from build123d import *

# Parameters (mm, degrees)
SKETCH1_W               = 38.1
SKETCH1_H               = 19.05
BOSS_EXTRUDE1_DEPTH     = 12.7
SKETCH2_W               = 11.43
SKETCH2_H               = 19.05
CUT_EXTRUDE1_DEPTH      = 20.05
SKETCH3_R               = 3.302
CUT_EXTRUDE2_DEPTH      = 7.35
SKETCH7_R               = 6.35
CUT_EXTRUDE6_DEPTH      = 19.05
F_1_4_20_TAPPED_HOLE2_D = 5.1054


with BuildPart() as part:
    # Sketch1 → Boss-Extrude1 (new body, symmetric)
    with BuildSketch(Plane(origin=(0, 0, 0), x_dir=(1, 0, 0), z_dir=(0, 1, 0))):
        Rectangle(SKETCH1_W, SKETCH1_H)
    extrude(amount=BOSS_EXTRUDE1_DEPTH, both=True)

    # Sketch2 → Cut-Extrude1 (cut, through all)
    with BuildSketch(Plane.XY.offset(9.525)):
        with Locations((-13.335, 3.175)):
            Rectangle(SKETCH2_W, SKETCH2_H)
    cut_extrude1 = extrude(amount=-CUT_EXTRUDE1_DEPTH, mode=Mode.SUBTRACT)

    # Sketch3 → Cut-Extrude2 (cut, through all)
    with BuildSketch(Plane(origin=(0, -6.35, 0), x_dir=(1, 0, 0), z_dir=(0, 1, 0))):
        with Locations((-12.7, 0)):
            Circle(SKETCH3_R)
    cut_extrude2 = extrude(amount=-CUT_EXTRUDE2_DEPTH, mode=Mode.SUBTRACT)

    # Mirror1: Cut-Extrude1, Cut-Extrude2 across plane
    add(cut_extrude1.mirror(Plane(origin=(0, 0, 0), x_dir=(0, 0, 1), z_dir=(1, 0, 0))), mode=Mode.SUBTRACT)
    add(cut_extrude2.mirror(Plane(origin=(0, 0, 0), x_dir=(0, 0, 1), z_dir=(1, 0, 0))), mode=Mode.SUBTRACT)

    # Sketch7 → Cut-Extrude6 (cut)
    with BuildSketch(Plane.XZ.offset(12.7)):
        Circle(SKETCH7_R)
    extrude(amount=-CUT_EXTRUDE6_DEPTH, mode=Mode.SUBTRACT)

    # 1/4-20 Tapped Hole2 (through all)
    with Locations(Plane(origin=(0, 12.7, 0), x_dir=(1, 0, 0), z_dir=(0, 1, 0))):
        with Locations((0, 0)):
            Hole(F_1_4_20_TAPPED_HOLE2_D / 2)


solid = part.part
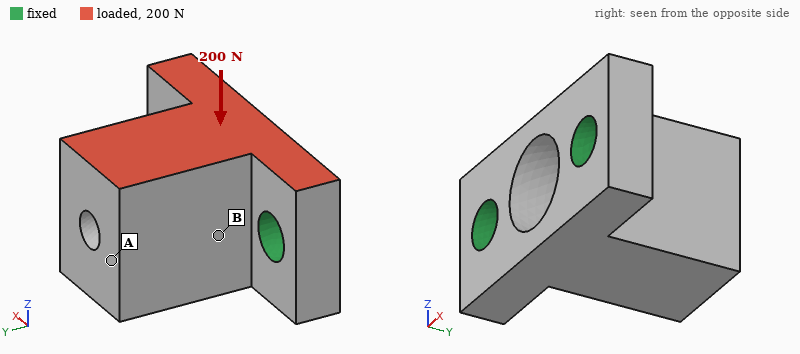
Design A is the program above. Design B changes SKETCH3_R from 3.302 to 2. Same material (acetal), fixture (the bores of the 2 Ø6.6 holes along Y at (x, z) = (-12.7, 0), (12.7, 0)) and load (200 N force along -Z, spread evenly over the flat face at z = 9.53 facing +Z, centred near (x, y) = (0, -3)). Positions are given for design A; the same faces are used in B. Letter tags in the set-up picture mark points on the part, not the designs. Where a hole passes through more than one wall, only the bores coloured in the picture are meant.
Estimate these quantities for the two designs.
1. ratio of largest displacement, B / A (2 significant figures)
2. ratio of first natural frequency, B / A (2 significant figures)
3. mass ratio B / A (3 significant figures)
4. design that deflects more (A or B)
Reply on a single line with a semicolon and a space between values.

1.4; 0.84; 1.04; B
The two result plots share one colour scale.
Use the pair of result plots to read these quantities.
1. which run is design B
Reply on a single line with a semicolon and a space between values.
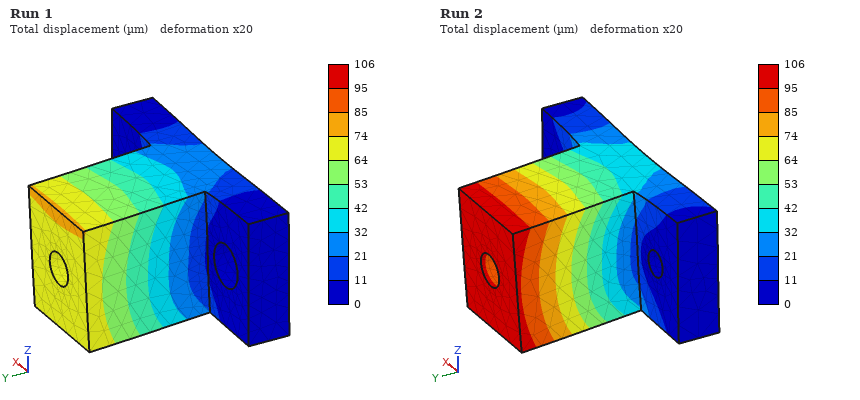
Run 2
